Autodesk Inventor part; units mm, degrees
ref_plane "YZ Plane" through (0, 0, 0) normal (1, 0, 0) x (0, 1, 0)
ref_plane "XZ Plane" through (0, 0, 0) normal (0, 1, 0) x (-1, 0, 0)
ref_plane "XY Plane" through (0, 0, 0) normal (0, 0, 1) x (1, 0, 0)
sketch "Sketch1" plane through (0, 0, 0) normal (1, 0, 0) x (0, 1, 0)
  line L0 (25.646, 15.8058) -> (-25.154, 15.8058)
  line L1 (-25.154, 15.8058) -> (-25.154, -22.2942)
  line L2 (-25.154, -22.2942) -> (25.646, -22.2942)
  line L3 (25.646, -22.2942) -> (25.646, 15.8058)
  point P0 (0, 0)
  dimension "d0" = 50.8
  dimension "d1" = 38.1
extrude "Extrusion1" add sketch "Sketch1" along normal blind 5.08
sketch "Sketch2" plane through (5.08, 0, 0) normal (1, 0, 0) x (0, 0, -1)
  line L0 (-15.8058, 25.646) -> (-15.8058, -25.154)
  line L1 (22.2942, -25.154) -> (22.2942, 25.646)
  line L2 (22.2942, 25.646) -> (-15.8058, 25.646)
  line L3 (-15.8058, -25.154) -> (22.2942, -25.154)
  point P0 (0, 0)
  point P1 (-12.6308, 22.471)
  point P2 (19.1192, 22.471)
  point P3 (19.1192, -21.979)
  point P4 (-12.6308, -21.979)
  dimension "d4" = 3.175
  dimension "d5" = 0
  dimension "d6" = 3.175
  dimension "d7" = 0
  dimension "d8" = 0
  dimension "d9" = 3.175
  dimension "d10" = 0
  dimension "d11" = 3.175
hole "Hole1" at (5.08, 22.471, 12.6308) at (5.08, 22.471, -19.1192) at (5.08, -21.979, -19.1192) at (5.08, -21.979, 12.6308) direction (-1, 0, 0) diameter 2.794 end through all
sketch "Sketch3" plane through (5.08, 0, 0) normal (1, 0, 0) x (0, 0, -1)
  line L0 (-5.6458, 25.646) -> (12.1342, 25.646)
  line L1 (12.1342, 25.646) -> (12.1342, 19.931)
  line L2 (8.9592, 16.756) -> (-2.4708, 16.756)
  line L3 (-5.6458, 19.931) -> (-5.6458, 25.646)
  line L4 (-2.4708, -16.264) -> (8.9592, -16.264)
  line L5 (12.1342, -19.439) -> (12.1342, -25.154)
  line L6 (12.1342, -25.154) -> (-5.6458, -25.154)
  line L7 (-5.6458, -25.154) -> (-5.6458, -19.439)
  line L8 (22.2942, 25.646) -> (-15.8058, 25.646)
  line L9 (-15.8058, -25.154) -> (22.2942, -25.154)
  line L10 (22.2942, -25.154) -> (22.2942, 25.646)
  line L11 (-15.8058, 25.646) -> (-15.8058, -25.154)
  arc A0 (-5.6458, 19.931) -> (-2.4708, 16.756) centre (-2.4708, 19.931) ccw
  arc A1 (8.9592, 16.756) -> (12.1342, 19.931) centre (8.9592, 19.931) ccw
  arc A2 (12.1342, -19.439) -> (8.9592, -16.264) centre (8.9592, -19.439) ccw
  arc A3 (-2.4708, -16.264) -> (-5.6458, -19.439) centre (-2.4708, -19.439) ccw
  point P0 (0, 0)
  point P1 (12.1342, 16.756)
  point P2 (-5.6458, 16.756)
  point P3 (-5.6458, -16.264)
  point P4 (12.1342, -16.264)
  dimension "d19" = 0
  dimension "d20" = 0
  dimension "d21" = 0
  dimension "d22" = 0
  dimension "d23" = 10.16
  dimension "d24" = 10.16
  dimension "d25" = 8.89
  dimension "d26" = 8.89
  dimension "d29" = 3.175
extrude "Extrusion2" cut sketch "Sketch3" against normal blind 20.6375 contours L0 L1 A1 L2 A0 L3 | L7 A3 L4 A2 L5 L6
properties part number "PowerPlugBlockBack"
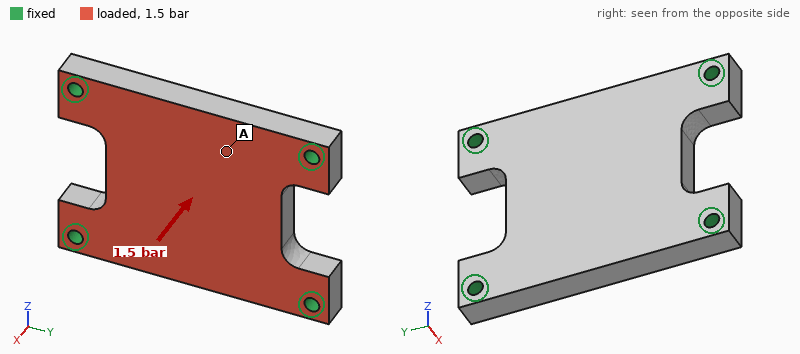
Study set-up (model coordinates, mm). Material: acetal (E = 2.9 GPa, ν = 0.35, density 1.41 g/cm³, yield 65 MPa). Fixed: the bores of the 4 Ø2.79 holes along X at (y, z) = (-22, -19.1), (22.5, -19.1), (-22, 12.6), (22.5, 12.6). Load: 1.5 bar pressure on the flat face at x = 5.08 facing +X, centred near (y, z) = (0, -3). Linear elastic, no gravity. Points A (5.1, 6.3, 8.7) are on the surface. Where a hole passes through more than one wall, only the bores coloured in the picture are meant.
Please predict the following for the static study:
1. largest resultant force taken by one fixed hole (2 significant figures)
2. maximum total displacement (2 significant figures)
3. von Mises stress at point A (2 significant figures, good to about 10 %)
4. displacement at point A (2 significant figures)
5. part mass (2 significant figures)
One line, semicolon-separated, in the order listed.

60 N; 90 µm; 2.8 MPa; 74 µm; 11 g
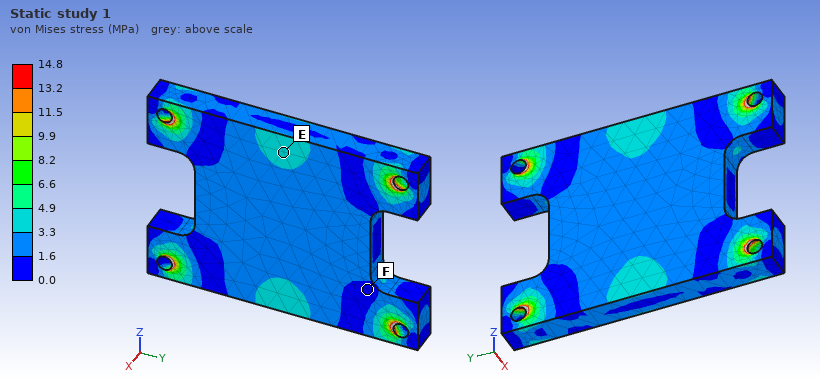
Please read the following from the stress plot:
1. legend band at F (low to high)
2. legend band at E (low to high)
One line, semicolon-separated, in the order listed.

0.0 to 1.6 MPa; 3.3 to 4.9 MPa
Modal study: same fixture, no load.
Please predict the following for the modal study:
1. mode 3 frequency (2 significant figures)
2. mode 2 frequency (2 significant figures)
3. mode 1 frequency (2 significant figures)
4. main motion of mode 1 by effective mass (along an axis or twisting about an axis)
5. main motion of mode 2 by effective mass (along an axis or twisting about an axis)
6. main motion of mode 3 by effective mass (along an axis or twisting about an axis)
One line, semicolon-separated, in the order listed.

6200 Hz; 4100 Hz; 2800 Hz; along X; twisting about Y; along Z
